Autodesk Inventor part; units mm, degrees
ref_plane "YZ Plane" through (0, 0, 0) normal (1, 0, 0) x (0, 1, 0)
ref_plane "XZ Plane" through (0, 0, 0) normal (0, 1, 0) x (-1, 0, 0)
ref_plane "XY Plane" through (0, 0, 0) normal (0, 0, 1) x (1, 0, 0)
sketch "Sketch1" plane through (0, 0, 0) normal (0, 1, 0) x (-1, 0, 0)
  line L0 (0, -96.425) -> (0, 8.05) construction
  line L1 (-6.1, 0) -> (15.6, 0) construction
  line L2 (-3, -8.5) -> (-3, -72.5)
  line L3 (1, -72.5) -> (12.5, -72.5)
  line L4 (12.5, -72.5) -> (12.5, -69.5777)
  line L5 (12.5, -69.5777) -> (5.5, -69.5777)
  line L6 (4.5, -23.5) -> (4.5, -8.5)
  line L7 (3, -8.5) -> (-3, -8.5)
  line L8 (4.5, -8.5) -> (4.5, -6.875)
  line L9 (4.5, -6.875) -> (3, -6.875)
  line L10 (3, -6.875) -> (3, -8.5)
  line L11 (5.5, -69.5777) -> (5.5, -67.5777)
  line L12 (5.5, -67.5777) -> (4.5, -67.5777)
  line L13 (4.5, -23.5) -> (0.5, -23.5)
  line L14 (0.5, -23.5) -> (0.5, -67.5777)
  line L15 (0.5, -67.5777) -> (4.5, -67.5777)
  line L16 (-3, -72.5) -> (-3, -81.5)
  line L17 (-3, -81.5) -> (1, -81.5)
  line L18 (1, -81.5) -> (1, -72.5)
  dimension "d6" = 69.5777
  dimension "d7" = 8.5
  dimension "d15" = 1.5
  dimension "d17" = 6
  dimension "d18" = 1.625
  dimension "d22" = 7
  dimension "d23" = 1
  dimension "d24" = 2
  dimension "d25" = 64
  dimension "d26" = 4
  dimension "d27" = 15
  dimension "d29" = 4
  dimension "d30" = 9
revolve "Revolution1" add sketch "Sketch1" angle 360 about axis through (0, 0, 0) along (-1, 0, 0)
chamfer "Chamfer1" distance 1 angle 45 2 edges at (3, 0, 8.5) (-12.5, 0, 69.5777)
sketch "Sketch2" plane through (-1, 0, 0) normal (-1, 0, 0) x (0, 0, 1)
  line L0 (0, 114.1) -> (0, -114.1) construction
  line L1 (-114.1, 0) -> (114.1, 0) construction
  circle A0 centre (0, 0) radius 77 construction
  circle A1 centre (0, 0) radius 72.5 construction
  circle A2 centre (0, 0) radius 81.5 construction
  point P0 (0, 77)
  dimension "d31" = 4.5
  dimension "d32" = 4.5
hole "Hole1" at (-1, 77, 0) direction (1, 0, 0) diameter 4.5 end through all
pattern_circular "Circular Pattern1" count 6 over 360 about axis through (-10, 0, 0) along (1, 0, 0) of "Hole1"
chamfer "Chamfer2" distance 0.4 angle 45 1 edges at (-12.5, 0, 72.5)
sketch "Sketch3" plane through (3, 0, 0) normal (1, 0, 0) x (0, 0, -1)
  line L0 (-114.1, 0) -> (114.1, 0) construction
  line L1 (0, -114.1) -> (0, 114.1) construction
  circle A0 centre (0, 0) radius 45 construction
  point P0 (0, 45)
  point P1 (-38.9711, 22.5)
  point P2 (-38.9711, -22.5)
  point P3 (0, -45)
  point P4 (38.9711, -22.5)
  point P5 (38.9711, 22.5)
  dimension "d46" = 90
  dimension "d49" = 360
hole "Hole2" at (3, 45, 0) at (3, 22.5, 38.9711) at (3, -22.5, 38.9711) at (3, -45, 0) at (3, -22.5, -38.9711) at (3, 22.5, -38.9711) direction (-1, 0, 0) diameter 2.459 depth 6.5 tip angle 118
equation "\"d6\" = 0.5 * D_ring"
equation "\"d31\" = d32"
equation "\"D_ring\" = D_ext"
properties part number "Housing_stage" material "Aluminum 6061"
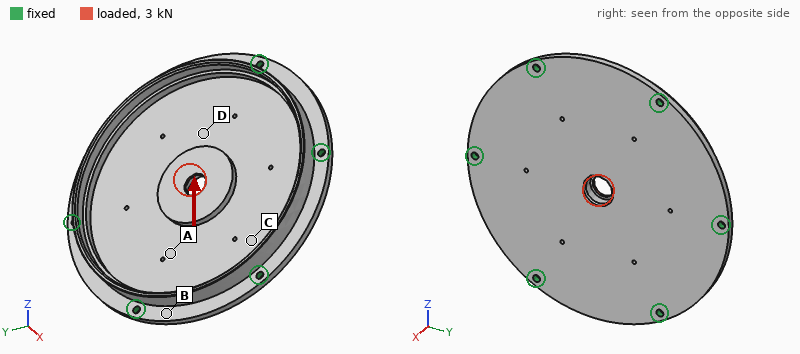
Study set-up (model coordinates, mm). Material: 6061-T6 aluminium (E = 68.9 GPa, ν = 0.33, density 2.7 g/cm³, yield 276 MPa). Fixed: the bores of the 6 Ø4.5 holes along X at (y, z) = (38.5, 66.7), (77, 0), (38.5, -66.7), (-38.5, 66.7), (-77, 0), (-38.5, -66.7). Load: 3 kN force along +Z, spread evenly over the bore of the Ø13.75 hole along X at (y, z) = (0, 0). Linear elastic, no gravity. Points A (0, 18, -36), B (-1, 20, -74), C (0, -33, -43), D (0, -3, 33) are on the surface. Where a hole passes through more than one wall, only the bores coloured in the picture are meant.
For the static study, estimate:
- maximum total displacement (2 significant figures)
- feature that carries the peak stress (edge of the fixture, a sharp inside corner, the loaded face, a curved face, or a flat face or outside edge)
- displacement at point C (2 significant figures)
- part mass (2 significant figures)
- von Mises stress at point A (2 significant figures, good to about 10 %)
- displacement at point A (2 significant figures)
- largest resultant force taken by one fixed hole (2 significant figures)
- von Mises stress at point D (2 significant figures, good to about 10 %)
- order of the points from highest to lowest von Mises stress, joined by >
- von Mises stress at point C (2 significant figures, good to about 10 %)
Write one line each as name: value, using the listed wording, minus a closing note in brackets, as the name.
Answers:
maximum total displacement: 45 µm
feature that carries the peak stress: the loaded face
displacement at point C: 16 µm
part mass: 270 g
von Mises stress at point A: 13 MPa
displacement at point A: 34 µm
largest resultant force taken by one fixed hole: 680 N
von Mises stress at point D: 20 MPa
order of the points from highest to lowest von Mises stress, joined by >: D > A > C > B
von Mises stress at point C: 7.6 MPa
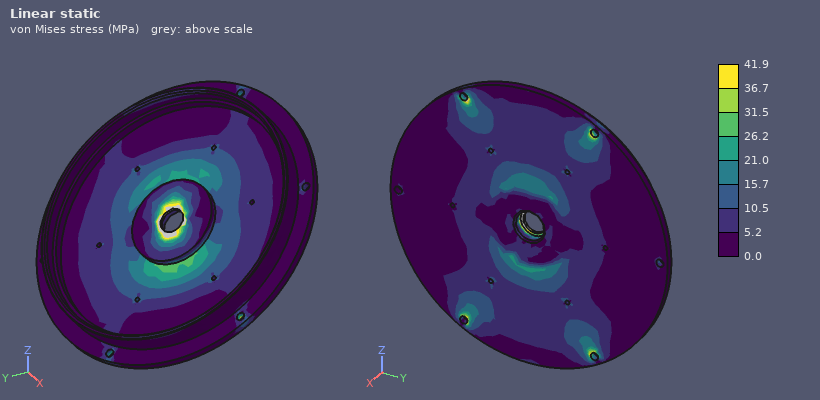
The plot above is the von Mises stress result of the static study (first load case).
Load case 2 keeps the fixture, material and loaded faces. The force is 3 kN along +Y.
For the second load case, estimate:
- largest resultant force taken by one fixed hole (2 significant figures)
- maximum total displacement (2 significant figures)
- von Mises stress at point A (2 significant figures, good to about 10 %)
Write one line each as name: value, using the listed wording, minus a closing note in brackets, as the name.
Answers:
largest resultant force taken by one fixed hole: 770 N
maximum total displacement: 45 µm
von Mises stress at point A: 10 MPa
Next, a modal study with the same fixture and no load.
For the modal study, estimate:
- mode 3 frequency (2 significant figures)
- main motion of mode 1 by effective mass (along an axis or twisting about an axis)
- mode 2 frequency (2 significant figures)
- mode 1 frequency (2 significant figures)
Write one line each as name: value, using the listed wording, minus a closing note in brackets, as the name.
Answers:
mode 3 frequency: 3000 Hz
main motion of mode 1 by effective mass: along X
mode 2 frequency: 3000 Hz
mode 1 frequency: 1500 Hz
